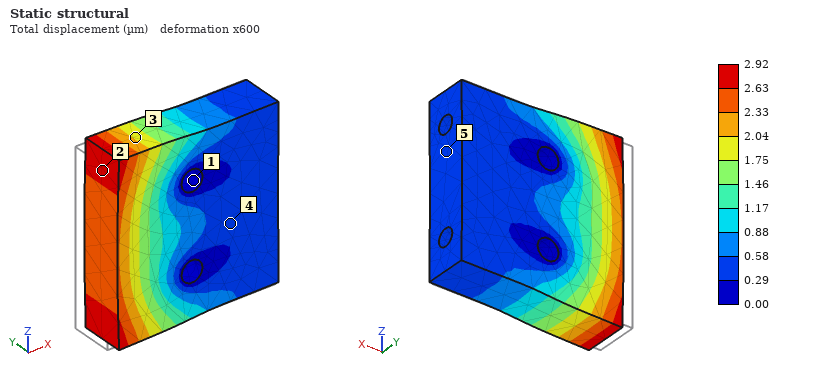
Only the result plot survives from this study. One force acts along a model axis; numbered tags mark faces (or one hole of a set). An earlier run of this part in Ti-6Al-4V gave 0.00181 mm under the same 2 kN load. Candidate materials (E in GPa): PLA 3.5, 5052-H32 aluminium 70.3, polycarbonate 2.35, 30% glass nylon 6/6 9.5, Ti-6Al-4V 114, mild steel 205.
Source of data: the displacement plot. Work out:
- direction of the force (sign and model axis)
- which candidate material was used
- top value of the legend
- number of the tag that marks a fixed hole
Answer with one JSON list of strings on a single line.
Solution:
["+X", "5052-H32 aluminium", "2.92 µm", "1"]
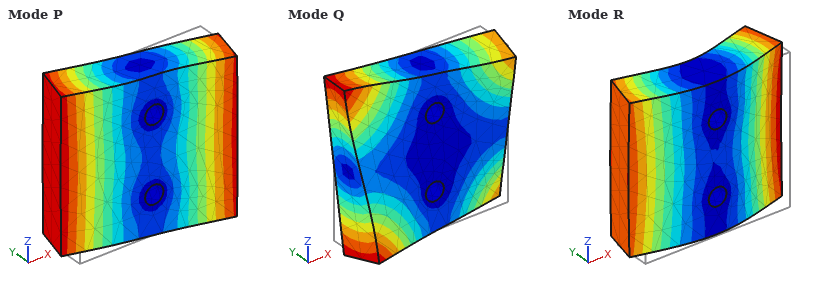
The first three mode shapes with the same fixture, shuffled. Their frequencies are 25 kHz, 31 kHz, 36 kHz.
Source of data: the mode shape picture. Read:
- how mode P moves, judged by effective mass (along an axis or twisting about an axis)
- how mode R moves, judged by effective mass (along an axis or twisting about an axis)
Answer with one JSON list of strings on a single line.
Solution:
["twisting about Z", "along Y"]
